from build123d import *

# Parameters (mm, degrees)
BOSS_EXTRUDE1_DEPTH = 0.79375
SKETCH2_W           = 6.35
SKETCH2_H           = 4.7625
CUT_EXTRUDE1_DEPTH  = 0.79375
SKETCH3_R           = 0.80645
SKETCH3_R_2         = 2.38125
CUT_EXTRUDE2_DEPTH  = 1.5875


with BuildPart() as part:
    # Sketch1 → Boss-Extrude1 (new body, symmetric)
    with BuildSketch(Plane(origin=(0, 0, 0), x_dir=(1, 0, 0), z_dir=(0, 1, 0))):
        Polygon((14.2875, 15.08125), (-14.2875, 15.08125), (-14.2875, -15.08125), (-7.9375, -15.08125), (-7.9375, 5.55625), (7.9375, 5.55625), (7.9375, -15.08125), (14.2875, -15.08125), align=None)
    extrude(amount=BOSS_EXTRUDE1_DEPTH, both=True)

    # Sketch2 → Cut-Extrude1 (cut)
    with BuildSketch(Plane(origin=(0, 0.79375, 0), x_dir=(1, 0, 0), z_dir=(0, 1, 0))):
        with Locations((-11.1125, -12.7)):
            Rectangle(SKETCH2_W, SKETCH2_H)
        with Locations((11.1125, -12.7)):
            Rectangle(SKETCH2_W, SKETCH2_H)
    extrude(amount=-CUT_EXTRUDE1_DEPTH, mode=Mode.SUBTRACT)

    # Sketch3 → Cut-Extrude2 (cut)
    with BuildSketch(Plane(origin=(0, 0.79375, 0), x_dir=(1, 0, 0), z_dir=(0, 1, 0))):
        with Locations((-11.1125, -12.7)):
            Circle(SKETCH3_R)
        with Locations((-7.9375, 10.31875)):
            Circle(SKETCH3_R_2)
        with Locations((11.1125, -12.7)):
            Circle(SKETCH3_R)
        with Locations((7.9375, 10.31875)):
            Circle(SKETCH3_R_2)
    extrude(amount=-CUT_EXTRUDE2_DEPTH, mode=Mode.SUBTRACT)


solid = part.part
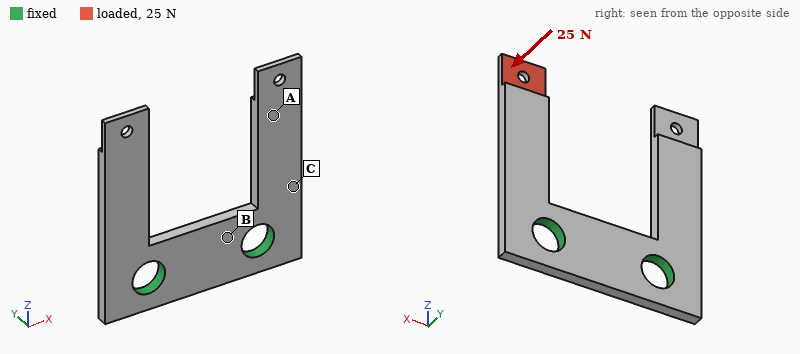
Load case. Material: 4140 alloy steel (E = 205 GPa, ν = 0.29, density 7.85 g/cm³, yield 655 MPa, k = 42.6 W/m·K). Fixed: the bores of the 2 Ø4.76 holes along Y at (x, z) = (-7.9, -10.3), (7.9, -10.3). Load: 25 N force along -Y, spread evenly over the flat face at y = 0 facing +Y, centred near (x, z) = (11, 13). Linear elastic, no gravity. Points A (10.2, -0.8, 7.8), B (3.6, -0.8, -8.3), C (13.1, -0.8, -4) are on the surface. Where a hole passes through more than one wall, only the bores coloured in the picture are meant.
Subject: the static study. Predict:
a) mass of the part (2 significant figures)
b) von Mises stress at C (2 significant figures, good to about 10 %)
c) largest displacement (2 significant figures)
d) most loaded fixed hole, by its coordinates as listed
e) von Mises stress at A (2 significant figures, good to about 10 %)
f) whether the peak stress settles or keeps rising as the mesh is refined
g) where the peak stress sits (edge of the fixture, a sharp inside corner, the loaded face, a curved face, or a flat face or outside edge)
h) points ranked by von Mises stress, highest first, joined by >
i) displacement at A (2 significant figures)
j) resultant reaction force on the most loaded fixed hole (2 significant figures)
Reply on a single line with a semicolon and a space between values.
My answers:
5.8 g; 150 MPa; 0.22 mm; (7.9, -10.3); 48 MPa; keeps rising; a sharp inside corner; C > A > B; 0.12 mm; 27 N
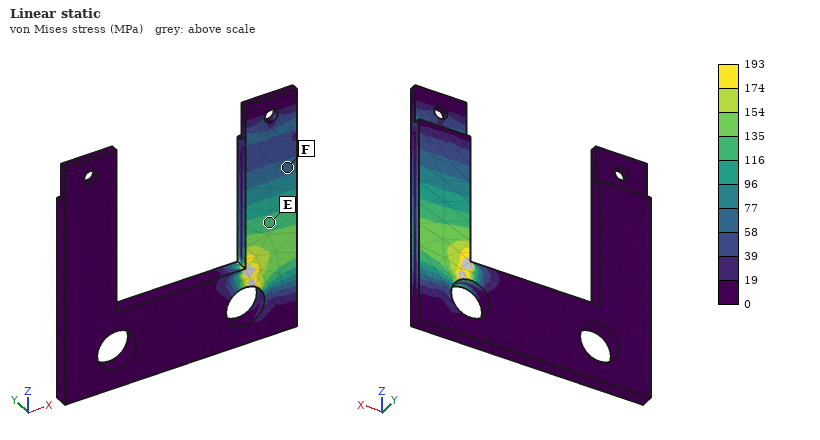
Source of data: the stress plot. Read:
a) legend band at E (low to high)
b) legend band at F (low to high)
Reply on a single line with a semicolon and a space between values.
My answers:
116 to 135 MPa; 58 to 77 MPa
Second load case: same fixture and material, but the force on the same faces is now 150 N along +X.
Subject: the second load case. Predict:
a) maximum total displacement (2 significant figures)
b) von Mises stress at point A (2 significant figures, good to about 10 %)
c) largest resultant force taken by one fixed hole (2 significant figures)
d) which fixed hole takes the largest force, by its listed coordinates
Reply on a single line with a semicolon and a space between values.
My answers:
94 µm; 34 MPa; 130 N; (7.9, -10.3)
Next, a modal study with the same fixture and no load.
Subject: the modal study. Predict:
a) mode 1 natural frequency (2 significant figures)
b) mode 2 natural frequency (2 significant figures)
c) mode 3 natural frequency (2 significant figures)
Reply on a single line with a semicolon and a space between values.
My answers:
2900 Hz; 2900 Hz; 10 kHz
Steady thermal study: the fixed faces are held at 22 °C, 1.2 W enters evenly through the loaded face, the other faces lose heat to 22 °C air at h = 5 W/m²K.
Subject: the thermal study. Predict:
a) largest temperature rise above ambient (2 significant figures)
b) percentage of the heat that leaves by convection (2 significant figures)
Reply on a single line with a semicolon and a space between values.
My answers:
68 K; 4.6 %
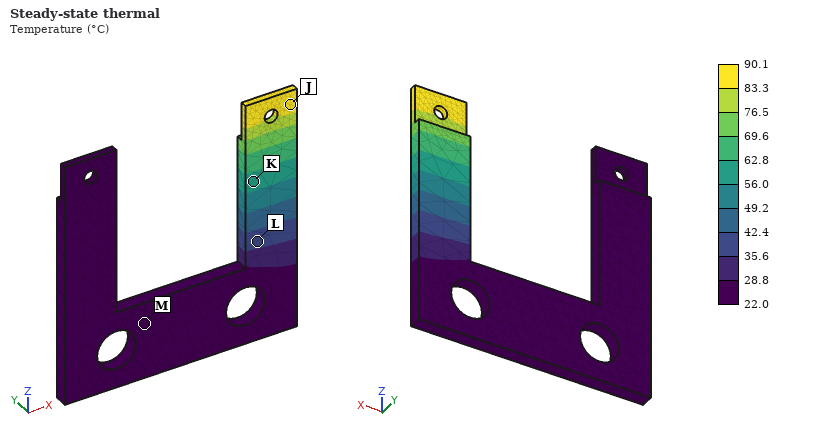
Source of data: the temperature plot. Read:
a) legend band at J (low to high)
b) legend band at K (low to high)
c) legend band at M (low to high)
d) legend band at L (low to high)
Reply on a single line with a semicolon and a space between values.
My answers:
83.3 to 90.1 °C; 56.0 to 62.8 °C; 22.0 to 28.8 °C; 35.6 to 42.4 °C
